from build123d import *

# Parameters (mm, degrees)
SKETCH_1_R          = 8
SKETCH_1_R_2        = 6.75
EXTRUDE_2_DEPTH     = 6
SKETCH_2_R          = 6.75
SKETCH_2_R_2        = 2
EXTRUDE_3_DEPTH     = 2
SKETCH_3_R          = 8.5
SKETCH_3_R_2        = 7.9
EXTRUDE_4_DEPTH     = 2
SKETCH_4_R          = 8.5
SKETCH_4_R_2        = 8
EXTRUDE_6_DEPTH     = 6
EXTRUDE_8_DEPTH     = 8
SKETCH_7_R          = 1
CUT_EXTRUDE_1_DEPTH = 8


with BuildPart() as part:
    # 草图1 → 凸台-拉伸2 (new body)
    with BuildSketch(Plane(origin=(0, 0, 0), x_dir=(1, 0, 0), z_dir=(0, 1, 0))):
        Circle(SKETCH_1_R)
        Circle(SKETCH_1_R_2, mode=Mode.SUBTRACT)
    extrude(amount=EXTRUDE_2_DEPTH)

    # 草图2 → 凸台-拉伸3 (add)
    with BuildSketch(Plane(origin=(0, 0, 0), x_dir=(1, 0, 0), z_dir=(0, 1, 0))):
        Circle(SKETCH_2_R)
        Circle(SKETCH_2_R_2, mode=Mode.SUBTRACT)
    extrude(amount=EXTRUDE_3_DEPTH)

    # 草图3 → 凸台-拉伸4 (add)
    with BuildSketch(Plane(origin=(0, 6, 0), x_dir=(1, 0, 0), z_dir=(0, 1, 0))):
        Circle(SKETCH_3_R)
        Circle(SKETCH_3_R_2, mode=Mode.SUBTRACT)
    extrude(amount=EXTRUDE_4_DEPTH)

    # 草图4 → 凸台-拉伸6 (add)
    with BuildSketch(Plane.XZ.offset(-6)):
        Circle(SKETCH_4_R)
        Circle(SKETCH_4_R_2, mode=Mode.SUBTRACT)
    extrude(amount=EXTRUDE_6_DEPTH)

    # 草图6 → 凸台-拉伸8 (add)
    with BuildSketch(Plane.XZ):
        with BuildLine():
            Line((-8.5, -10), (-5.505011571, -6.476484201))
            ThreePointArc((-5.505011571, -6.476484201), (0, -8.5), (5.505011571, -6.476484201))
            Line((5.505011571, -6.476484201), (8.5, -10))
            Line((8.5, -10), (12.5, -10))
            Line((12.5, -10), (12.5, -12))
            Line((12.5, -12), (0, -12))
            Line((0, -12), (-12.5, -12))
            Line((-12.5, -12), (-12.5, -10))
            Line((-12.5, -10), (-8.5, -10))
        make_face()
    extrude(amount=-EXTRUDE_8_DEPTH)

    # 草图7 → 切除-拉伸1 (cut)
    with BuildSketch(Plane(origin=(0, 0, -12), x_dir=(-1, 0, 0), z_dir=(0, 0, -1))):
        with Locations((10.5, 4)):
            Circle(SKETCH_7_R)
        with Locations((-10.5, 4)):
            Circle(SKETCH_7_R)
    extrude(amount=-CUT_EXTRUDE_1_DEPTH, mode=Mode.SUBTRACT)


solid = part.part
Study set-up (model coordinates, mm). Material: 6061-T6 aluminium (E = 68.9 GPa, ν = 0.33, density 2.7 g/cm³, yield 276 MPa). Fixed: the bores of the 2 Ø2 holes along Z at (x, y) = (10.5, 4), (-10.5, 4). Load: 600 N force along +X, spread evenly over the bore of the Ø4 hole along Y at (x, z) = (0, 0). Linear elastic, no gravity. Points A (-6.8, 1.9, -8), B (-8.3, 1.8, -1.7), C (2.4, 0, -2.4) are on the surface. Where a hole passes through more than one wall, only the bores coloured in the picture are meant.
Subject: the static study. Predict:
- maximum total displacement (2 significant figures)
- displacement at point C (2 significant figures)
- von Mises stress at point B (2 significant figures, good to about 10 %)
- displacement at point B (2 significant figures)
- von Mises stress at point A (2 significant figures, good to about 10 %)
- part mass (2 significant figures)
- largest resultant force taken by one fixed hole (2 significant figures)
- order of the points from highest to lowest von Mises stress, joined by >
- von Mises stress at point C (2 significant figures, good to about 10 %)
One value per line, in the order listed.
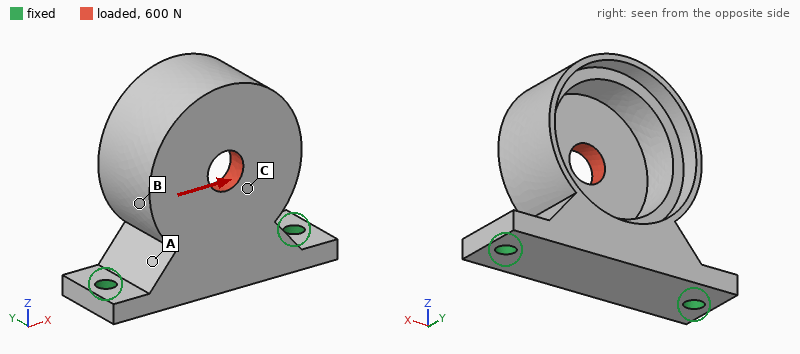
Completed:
50 µm
17 µm
15 MPa
27 µm
73 MPa
4.0 g
480 N
A > C > B
38 MPa
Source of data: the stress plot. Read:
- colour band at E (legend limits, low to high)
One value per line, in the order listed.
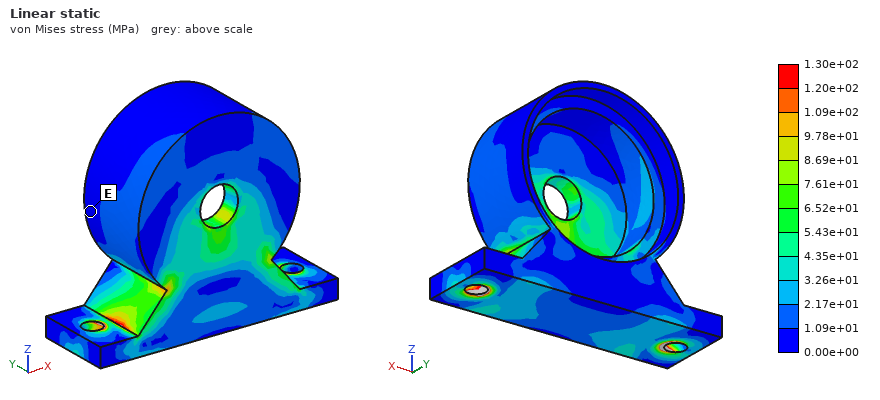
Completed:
0.00e+00 to 1.09e+01 MPa
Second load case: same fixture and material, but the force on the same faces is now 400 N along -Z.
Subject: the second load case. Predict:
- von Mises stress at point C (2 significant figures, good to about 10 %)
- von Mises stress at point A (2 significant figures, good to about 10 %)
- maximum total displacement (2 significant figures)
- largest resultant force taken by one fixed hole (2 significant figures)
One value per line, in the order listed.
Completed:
21 MPa
44 MPa
67 µm
250 N
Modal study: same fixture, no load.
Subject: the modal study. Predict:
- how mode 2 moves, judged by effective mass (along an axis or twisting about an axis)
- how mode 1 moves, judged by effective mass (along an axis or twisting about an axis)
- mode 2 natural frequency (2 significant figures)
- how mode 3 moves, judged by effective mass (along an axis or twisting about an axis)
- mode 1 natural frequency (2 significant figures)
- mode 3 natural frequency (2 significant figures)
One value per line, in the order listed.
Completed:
along X
along Y
12 kHz
along Z
4900 Hz
19 kHz
